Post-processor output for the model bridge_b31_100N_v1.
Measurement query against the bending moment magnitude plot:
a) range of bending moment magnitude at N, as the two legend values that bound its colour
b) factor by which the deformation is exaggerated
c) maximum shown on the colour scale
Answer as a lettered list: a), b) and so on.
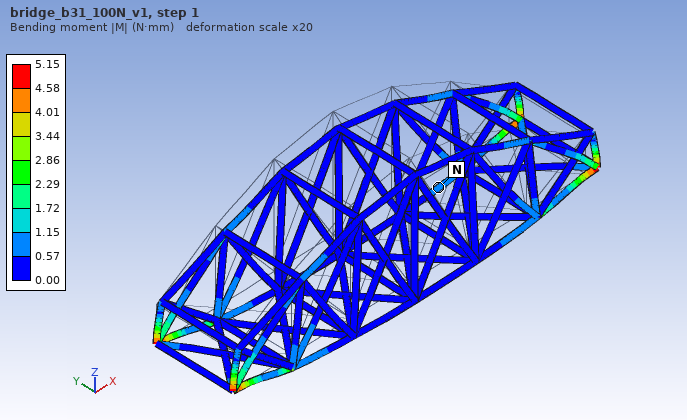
a) 0.57 to 1.15 N·mm
b) 20
c) 5.15 N·mm
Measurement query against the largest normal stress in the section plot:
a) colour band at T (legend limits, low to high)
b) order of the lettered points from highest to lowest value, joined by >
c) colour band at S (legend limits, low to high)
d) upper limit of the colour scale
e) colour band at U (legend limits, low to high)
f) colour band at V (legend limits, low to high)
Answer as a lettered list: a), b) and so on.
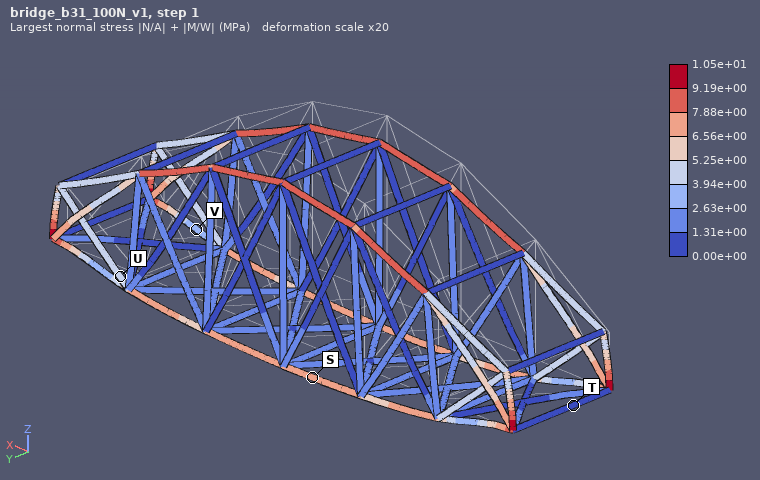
a) 0.00e+00 to 1.31e+00 MPa
b) S > U > V > T
c) 6.56e+00 to 7.88e+00 MPa
d) 1.05e+01 MPa
e) 3.94e+00 to 5.25e+00 MPa
f) 2.63e+00 to 3.94e+00 MPa
